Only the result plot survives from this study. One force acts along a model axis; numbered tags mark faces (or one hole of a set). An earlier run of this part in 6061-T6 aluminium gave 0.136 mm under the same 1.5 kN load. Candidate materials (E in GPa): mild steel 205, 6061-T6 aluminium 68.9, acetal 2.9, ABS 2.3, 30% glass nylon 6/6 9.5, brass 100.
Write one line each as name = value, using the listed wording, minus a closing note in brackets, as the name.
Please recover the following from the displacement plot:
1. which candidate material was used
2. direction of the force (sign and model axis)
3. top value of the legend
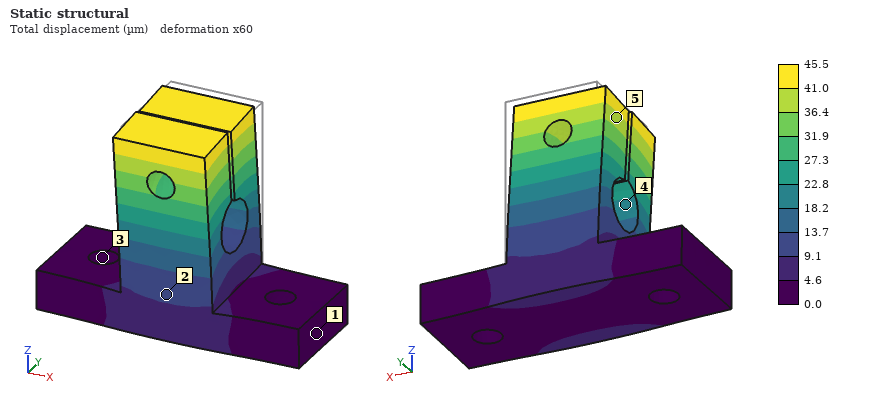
which candidate material was used = mild steel
direction of the force = -Y
top value of the legend = 45.5 µm
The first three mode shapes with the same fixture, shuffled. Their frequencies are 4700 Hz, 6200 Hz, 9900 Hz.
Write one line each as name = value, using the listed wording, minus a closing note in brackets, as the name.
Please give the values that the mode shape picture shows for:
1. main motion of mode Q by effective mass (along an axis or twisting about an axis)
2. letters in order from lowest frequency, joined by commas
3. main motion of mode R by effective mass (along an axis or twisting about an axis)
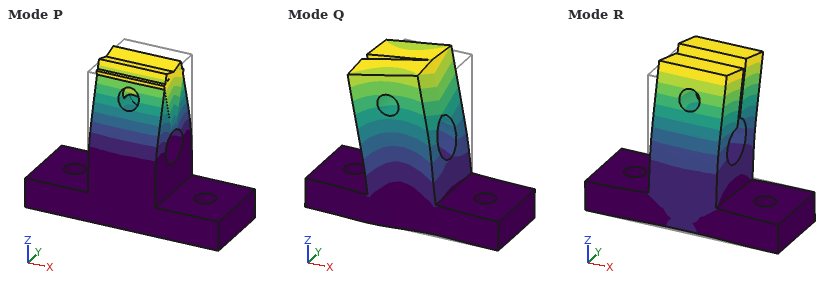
main motion of mode Q by effective mass = along X
letters in order from lowest frequency, joined by commas = R, P, Q
main motion of mode R by effective mass = along Y
